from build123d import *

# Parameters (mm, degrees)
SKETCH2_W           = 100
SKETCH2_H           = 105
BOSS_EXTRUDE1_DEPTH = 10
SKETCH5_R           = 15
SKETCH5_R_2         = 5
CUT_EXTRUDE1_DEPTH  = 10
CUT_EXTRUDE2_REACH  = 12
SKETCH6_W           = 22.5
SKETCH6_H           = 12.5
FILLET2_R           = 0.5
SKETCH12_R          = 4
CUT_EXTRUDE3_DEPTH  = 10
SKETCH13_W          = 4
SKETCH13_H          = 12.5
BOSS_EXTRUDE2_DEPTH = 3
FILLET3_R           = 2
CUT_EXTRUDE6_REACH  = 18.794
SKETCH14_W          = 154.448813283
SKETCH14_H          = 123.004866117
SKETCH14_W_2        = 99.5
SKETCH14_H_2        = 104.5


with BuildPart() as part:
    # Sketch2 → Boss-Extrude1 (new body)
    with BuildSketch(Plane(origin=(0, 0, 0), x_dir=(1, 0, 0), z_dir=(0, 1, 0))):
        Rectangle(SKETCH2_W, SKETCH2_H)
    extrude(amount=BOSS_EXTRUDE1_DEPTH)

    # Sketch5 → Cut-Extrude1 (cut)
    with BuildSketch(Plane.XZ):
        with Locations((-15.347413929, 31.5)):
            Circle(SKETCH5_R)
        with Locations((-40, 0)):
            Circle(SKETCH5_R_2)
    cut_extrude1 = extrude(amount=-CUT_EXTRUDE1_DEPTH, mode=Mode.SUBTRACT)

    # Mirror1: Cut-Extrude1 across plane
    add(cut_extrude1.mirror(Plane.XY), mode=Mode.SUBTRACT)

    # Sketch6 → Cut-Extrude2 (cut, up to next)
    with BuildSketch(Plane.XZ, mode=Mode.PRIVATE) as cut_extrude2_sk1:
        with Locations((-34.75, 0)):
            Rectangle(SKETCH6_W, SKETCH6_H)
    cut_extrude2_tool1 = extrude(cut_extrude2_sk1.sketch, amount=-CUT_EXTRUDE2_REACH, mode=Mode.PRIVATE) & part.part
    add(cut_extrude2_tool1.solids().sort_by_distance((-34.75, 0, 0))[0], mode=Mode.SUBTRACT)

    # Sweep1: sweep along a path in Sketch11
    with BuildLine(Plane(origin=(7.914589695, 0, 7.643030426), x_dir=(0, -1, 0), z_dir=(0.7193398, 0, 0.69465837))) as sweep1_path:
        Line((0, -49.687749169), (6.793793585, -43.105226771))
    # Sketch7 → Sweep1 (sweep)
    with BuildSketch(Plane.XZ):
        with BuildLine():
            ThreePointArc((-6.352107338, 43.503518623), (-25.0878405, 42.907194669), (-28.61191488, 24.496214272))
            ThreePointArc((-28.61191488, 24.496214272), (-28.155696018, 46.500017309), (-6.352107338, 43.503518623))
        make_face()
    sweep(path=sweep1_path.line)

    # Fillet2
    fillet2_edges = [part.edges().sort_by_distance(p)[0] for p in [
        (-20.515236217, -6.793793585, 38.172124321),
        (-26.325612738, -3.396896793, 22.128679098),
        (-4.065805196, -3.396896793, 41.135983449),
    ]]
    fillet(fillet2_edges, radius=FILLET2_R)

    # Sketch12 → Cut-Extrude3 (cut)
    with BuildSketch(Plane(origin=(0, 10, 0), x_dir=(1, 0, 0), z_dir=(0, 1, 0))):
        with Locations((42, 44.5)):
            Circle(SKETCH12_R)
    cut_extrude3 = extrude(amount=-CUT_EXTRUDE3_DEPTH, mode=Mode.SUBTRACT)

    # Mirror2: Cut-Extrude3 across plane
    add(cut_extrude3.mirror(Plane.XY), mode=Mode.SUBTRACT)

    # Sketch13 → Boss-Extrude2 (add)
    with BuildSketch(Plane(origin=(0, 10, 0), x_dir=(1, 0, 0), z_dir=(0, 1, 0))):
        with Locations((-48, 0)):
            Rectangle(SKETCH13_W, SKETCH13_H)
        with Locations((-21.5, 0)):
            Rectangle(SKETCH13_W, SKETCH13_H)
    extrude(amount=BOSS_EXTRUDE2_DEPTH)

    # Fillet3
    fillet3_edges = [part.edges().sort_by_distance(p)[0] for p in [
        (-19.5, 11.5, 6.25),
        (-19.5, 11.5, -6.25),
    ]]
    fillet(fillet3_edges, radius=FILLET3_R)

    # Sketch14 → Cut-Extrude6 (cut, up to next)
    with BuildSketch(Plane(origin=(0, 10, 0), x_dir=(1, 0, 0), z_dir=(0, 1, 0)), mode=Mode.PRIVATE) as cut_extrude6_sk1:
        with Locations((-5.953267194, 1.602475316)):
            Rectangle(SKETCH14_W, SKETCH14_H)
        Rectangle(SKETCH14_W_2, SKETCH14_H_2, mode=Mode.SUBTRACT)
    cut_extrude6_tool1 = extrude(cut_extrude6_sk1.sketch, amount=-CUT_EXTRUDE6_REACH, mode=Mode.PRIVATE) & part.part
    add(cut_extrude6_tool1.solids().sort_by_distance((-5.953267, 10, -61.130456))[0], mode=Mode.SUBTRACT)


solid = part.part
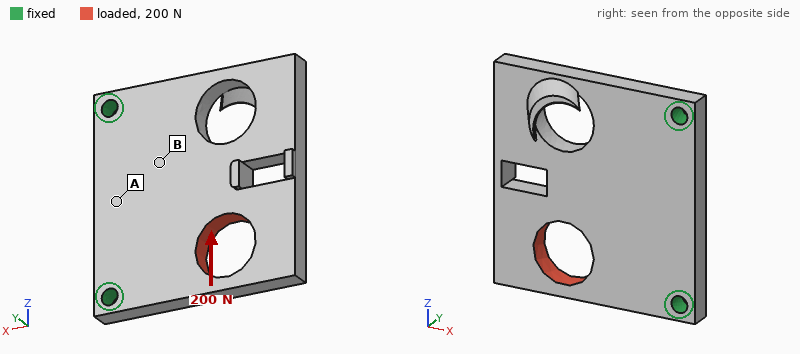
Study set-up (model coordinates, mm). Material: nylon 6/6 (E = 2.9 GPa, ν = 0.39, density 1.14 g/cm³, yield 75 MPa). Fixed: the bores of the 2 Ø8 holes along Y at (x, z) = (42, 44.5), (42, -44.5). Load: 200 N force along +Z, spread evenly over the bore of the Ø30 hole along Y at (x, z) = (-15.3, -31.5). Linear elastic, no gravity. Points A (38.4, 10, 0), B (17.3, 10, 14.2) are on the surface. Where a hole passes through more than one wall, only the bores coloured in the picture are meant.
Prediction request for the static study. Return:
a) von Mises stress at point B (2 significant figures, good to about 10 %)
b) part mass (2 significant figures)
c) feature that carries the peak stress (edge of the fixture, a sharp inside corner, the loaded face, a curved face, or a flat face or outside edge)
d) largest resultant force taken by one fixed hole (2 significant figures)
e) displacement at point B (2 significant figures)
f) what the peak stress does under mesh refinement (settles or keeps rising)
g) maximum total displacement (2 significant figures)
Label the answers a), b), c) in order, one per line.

a) 0.37 MPa
b) 99 g
c) edge of the fixture
d) 160 N
e) 7.2 µm
f) keeps rising
g) 42 µm
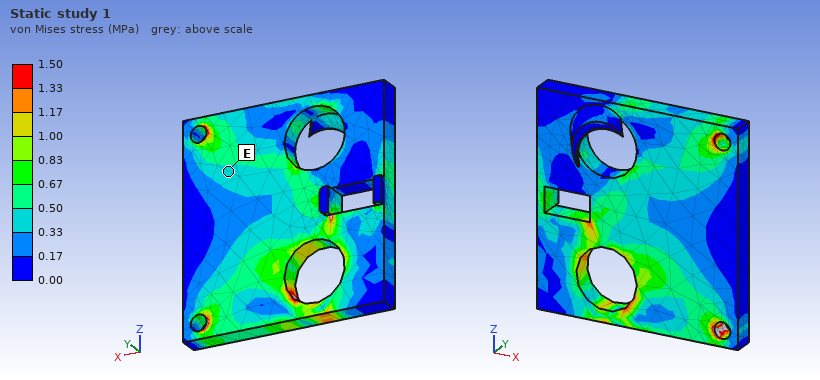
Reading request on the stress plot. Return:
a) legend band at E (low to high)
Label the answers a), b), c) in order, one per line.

a) 0.33 to 0.50 MPa
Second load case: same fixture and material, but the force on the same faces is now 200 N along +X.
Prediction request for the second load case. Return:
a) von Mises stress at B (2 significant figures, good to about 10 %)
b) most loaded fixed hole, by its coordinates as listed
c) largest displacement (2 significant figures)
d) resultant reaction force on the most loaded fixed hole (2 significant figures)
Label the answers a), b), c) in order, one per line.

a) 0.15 MPa
b) (42, -44.5)
c) 23 µm
d) 170 N
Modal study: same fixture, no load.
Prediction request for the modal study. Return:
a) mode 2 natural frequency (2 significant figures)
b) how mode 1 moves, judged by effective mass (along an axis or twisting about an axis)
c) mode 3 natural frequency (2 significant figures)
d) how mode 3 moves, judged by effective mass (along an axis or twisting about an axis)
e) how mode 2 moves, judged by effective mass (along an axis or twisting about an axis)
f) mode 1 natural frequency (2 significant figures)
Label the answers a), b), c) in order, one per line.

a) 610 Hz
b) along Y
c) 1300 Hz
d) along Y
e) twisting about X
f) 270 Hz
